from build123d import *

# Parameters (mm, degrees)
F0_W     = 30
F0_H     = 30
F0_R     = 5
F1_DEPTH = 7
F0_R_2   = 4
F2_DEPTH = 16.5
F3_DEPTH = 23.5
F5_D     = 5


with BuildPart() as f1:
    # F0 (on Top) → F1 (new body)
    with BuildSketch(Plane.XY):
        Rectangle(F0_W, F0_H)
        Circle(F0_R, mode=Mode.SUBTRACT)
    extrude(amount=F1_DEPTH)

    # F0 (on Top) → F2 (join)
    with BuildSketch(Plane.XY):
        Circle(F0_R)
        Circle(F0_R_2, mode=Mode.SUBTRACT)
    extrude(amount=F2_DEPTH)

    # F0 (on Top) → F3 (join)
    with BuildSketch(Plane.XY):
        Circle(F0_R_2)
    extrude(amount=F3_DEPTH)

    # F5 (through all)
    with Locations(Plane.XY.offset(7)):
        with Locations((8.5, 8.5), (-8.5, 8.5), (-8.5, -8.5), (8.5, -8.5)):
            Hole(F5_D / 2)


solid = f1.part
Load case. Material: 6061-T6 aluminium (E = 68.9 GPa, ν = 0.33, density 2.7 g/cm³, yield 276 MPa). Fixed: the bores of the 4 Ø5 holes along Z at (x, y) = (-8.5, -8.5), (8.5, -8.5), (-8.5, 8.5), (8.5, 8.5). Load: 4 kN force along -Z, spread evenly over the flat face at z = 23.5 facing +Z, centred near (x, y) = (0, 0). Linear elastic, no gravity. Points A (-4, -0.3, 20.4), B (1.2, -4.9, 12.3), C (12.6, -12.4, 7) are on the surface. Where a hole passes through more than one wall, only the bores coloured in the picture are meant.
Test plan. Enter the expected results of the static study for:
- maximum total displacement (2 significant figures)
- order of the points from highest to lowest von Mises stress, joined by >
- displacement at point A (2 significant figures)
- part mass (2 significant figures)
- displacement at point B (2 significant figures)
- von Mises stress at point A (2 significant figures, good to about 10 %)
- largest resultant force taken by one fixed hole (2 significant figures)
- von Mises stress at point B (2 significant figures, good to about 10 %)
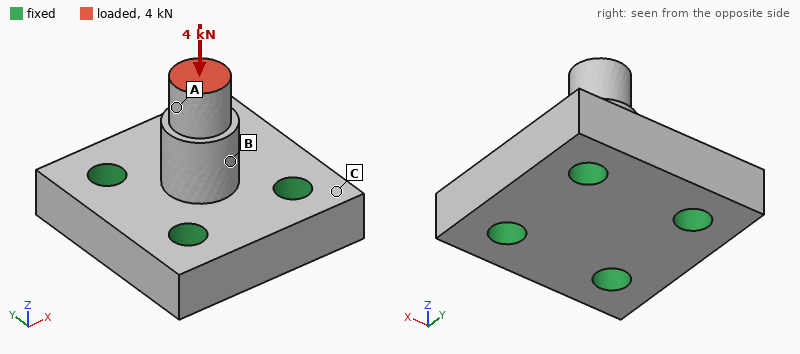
22 µm
A > B > C
18 µm
18 g
10 µm
79 MPa
1.0 kN
47 MPa
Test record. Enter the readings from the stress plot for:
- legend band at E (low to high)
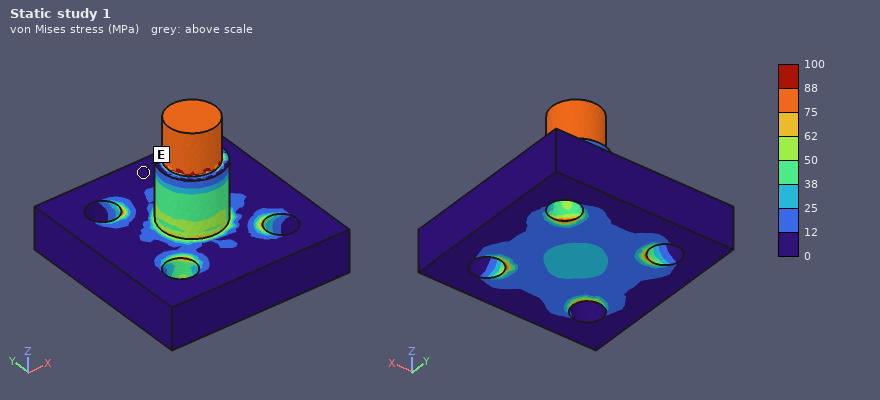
0 to 12 MPa
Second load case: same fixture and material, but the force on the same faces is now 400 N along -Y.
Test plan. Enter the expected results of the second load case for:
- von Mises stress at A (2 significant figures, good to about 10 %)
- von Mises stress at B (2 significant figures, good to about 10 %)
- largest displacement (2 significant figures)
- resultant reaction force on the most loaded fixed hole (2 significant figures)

16 MPa
43 MPa
36 µm
290 N
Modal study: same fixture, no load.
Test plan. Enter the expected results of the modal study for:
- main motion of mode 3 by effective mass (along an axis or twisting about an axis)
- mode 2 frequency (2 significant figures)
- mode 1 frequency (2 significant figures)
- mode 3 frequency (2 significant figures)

along Z
21 kHz
20 kHz
49 kHz
